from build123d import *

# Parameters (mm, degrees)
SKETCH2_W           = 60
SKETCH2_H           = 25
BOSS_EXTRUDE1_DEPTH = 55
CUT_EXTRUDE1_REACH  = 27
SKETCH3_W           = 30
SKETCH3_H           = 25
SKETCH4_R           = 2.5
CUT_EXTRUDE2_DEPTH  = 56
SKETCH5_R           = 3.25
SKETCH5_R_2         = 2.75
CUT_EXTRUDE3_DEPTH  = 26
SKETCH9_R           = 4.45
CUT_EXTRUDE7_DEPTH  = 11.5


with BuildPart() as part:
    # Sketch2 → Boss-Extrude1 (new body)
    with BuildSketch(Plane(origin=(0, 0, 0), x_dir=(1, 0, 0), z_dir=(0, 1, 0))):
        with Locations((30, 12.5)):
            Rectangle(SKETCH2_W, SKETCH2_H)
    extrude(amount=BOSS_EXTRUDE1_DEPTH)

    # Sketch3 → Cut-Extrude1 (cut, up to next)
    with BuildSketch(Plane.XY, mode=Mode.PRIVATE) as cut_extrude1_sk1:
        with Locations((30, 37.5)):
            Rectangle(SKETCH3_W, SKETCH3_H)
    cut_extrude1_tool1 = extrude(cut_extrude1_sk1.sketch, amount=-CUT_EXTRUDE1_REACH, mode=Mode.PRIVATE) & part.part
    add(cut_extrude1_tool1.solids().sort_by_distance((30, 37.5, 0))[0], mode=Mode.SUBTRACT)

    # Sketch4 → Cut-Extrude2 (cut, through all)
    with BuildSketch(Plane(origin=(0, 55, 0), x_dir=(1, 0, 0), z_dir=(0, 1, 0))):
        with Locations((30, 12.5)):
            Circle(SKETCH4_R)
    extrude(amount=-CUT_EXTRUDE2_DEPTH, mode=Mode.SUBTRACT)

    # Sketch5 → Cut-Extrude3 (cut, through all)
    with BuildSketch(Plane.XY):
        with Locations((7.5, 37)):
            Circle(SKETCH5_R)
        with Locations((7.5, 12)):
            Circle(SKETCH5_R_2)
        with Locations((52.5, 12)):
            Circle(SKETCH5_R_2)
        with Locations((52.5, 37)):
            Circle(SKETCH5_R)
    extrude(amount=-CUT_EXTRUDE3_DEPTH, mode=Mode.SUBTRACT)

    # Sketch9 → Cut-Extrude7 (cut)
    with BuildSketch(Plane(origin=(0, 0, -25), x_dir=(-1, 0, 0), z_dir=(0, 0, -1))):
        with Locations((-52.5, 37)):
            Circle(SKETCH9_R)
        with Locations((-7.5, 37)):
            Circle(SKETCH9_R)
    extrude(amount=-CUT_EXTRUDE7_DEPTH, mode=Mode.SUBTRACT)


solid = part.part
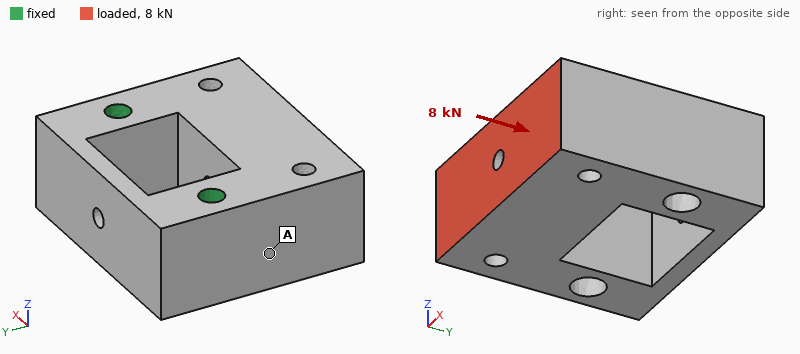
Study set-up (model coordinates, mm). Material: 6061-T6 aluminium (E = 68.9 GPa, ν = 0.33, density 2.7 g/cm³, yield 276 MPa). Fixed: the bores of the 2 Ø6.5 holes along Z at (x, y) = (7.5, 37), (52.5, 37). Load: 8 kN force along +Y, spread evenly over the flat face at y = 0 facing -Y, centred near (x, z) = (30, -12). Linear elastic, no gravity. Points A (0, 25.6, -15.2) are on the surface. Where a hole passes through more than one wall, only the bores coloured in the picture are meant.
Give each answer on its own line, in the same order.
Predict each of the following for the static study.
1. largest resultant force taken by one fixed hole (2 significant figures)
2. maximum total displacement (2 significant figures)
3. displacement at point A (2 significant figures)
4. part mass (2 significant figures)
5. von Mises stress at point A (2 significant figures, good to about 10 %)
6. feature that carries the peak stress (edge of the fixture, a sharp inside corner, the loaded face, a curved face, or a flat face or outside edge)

4.1 kN
20 µm
6.2 µm
160 g
8.9 MPa
edge of the fixture
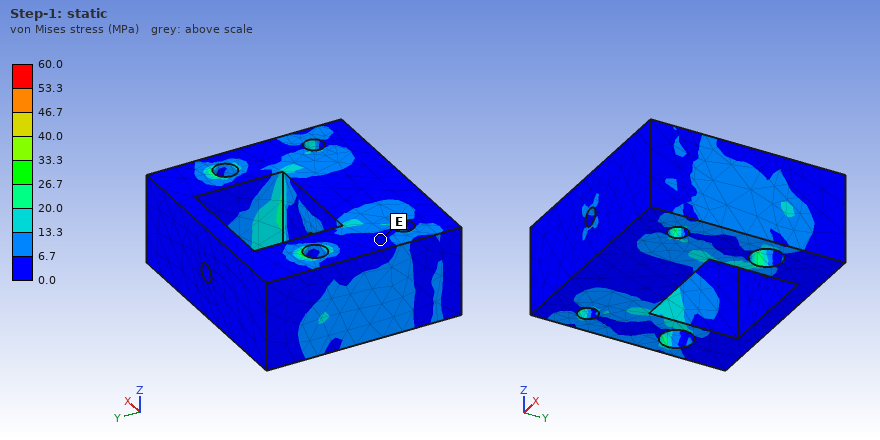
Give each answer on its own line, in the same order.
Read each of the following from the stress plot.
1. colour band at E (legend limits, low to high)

0.0 to 6.7 MPa
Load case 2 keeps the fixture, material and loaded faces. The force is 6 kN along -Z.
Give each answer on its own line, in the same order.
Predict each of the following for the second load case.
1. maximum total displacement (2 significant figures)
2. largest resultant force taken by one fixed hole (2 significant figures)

0.11 mm
3.0 kN
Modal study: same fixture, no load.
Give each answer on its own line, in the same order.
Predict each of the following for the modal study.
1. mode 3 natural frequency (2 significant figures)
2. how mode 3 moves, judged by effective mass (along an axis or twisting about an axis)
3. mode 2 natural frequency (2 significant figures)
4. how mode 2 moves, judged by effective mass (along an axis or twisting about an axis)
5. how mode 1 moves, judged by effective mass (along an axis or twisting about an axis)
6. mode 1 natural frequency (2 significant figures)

11 kHz
twisting about Y
9800 Hz
along X
along Z
5600 Hz
